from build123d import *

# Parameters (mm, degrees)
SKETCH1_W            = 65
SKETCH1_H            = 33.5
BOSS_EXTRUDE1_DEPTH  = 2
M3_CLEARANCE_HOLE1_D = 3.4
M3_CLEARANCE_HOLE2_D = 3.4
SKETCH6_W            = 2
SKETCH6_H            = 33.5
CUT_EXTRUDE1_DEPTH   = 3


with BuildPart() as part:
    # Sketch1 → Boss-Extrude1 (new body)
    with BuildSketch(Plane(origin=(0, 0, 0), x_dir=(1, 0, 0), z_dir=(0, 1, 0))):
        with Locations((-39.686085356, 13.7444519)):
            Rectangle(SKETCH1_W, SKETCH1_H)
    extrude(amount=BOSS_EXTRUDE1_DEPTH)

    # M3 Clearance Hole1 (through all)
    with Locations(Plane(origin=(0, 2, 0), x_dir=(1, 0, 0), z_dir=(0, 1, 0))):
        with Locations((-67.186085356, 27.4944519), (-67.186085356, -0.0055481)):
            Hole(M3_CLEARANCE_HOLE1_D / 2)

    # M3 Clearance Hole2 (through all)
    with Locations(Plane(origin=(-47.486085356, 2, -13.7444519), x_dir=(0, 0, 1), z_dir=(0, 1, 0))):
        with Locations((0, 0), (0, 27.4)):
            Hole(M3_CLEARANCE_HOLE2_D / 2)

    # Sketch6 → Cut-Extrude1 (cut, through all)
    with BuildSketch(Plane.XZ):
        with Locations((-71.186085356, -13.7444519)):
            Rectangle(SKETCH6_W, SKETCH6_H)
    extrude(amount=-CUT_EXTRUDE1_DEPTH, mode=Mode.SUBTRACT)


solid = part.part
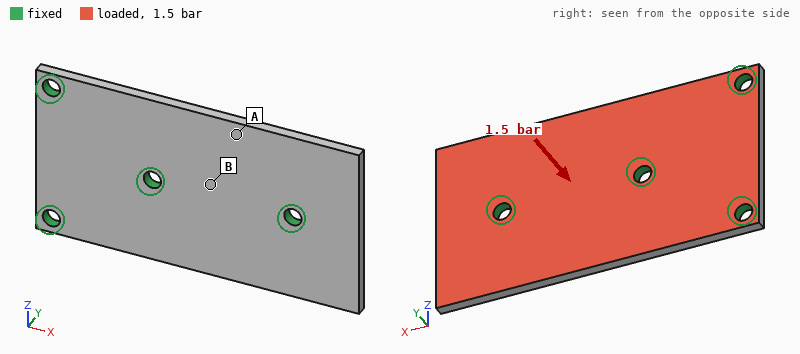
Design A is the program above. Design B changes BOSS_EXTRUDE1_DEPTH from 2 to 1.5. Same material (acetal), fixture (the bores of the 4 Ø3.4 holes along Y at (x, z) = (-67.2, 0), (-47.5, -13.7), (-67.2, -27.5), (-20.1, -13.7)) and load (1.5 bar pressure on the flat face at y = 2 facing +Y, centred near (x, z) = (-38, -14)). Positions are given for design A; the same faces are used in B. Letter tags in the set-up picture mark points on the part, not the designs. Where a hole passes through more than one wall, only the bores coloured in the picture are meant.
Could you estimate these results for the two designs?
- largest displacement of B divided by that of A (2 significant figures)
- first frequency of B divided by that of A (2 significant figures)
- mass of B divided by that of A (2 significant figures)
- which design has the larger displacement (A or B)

2.3
0.77
0.75
B
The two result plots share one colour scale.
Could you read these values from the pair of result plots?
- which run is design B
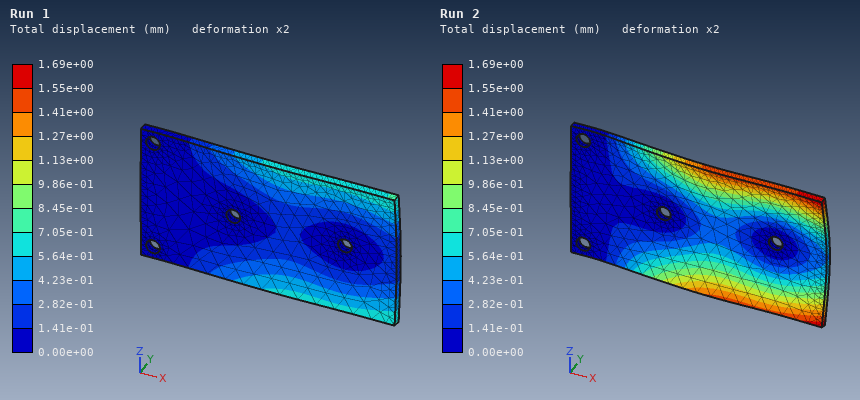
Run 2
